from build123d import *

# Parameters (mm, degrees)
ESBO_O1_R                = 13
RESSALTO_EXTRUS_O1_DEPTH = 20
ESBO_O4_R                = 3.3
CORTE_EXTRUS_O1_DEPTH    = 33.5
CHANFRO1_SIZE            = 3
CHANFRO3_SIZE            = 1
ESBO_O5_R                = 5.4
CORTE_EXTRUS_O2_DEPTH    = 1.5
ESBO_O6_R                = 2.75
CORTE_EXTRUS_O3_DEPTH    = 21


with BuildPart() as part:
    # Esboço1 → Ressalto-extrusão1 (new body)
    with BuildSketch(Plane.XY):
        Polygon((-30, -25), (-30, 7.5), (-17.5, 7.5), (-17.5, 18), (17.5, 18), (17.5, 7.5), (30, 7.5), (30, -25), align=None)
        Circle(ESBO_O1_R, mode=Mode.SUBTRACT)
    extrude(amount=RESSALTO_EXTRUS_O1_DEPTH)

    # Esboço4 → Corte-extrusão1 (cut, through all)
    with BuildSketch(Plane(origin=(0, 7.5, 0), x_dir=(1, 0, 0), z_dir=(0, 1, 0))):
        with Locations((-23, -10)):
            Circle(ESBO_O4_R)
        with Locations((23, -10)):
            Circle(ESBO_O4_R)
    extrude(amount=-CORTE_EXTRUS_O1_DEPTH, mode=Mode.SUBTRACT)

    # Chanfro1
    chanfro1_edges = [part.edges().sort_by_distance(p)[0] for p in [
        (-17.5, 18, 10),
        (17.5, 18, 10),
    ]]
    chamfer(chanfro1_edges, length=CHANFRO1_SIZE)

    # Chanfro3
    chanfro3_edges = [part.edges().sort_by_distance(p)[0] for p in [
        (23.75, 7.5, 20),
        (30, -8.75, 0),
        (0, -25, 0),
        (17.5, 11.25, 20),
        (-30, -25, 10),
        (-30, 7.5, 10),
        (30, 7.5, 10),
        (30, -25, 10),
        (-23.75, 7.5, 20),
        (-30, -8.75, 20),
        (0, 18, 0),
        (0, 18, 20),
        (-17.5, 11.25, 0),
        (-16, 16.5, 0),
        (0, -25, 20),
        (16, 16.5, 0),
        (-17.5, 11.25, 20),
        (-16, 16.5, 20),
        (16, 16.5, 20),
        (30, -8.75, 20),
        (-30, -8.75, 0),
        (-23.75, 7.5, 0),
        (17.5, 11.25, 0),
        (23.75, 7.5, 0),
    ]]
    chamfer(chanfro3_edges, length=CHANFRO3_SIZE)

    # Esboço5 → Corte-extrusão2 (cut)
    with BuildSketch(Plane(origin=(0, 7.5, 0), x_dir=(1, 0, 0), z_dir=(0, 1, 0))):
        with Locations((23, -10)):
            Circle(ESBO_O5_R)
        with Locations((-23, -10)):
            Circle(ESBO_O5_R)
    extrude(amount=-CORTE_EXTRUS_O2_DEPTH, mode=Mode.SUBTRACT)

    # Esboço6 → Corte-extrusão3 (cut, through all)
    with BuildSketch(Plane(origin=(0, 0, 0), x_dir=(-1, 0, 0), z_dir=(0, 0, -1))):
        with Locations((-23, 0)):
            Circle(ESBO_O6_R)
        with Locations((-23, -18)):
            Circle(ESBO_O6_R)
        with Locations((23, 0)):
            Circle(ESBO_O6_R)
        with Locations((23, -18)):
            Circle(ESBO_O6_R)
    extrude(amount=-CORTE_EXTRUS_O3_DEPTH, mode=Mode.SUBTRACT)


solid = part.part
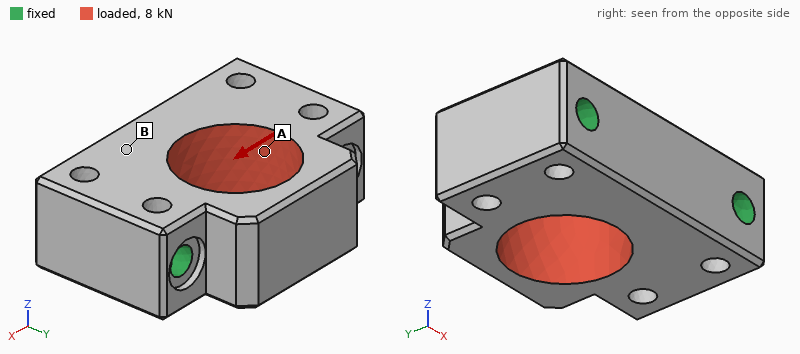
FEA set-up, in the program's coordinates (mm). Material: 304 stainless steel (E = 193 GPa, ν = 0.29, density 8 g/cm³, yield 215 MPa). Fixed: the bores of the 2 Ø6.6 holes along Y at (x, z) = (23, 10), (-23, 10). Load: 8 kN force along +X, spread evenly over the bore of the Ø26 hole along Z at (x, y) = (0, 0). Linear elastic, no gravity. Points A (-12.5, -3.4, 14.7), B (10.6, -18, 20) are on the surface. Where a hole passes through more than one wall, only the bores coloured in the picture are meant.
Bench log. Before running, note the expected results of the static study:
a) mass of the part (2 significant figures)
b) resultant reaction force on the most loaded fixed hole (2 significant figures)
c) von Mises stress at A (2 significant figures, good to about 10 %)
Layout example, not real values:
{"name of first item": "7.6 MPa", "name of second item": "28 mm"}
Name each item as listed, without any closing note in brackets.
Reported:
{"mass of the part": "250 g", "resultant reaction force on the most loaded fixed hole": "4.0 kN", "von Mises stress at A": "10 MPa"}
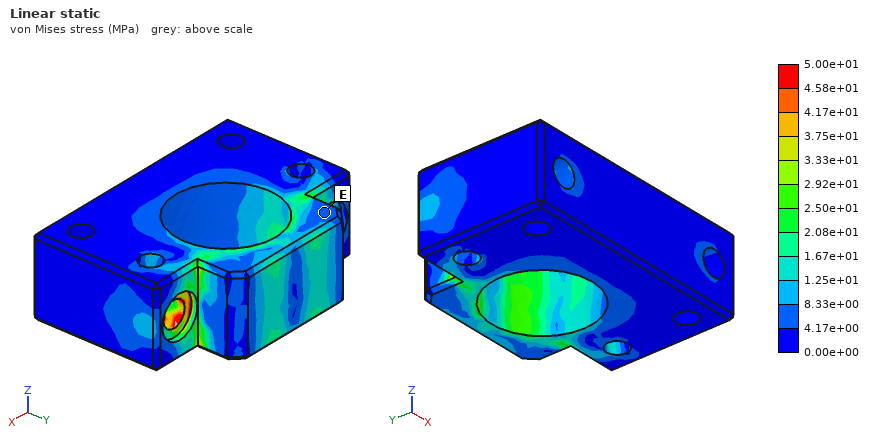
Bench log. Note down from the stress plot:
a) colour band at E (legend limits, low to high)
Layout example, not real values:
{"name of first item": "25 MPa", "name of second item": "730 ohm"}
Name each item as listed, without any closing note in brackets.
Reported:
{"colour band at E": "4.17e+00 to 8.33e+00 MPa"}
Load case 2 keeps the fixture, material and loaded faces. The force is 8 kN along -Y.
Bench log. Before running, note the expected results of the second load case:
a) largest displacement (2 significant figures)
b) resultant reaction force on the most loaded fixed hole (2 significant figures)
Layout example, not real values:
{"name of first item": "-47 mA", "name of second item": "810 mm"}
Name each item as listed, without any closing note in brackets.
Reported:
{"largest displacement": "3.5 µm", "resultant reaction force on the most loaded fixed hole": "4.1 kN"}
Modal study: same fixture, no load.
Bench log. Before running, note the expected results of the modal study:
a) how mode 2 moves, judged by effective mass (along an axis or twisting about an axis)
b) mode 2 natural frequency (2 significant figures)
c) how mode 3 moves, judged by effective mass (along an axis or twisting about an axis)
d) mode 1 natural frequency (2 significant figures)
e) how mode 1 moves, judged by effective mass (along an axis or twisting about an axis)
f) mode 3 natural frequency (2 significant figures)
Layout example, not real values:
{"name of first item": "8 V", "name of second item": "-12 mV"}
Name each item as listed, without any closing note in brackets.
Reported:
{"how mode 2 moves, judged by effective mass": "along X", "mode 2 natural frequency": "23 kHz", "how mode 3 moves, judged by effective mass": "along Z", "mode 1 natural frequency": "16 kHz", "how mode 1 moves, judged by effective mass": "along Z", "mode 3 natural frequency": "25 kHz"}
